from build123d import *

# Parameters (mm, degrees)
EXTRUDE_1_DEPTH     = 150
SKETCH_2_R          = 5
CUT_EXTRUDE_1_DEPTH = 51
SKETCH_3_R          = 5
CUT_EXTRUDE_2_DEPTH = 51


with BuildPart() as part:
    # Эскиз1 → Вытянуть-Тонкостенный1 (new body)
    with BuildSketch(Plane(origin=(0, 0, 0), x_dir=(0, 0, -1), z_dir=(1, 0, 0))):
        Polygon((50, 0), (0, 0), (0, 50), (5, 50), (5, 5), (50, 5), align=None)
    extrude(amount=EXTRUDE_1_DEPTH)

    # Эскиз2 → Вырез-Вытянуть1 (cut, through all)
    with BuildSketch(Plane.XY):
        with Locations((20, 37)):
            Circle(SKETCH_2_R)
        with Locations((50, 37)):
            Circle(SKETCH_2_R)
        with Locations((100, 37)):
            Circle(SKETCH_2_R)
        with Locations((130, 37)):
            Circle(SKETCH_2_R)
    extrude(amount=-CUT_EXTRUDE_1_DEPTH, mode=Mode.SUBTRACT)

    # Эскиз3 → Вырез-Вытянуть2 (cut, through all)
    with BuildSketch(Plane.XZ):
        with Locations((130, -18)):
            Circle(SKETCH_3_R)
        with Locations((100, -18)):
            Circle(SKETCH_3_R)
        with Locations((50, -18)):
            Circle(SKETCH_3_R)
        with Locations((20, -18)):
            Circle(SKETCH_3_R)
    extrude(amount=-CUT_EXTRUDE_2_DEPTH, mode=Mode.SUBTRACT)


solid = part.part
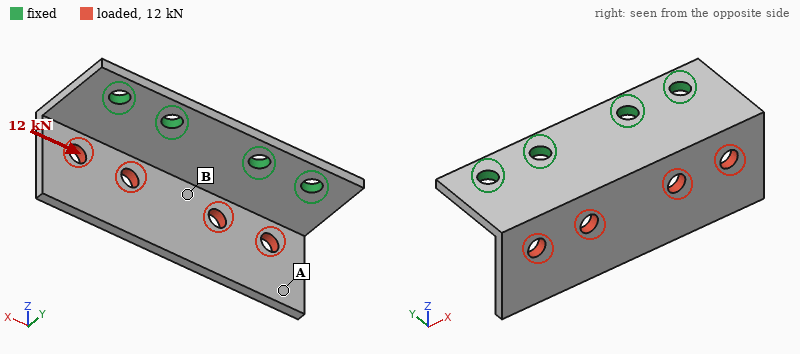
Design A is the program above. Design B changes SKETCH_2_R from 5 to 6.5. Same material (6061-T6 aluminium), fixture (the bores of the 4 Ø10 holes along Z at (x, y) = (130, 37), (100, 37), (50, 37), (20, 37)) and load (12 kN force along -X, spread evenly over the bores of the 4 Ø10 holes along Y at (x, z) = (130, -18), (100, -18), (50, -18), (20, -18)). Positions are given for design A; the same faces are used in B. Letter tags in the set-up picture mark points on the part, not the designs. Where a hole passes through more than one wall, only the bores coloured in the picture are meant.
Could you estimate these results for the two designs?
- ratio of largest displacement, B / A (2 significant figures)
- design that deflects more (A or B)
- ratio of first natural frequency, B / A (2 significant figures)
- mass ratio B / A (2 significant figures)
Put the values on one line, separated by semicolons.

0.90; A; 1.0; 0.98
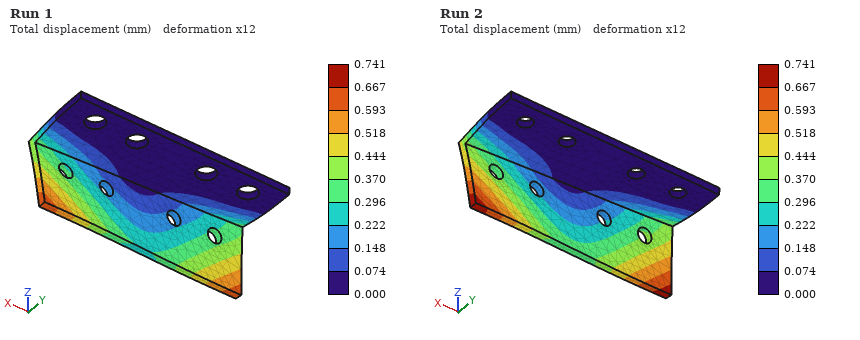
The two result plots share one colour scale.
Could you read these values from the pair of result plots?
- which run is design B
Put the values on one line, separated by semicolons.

Run 1
